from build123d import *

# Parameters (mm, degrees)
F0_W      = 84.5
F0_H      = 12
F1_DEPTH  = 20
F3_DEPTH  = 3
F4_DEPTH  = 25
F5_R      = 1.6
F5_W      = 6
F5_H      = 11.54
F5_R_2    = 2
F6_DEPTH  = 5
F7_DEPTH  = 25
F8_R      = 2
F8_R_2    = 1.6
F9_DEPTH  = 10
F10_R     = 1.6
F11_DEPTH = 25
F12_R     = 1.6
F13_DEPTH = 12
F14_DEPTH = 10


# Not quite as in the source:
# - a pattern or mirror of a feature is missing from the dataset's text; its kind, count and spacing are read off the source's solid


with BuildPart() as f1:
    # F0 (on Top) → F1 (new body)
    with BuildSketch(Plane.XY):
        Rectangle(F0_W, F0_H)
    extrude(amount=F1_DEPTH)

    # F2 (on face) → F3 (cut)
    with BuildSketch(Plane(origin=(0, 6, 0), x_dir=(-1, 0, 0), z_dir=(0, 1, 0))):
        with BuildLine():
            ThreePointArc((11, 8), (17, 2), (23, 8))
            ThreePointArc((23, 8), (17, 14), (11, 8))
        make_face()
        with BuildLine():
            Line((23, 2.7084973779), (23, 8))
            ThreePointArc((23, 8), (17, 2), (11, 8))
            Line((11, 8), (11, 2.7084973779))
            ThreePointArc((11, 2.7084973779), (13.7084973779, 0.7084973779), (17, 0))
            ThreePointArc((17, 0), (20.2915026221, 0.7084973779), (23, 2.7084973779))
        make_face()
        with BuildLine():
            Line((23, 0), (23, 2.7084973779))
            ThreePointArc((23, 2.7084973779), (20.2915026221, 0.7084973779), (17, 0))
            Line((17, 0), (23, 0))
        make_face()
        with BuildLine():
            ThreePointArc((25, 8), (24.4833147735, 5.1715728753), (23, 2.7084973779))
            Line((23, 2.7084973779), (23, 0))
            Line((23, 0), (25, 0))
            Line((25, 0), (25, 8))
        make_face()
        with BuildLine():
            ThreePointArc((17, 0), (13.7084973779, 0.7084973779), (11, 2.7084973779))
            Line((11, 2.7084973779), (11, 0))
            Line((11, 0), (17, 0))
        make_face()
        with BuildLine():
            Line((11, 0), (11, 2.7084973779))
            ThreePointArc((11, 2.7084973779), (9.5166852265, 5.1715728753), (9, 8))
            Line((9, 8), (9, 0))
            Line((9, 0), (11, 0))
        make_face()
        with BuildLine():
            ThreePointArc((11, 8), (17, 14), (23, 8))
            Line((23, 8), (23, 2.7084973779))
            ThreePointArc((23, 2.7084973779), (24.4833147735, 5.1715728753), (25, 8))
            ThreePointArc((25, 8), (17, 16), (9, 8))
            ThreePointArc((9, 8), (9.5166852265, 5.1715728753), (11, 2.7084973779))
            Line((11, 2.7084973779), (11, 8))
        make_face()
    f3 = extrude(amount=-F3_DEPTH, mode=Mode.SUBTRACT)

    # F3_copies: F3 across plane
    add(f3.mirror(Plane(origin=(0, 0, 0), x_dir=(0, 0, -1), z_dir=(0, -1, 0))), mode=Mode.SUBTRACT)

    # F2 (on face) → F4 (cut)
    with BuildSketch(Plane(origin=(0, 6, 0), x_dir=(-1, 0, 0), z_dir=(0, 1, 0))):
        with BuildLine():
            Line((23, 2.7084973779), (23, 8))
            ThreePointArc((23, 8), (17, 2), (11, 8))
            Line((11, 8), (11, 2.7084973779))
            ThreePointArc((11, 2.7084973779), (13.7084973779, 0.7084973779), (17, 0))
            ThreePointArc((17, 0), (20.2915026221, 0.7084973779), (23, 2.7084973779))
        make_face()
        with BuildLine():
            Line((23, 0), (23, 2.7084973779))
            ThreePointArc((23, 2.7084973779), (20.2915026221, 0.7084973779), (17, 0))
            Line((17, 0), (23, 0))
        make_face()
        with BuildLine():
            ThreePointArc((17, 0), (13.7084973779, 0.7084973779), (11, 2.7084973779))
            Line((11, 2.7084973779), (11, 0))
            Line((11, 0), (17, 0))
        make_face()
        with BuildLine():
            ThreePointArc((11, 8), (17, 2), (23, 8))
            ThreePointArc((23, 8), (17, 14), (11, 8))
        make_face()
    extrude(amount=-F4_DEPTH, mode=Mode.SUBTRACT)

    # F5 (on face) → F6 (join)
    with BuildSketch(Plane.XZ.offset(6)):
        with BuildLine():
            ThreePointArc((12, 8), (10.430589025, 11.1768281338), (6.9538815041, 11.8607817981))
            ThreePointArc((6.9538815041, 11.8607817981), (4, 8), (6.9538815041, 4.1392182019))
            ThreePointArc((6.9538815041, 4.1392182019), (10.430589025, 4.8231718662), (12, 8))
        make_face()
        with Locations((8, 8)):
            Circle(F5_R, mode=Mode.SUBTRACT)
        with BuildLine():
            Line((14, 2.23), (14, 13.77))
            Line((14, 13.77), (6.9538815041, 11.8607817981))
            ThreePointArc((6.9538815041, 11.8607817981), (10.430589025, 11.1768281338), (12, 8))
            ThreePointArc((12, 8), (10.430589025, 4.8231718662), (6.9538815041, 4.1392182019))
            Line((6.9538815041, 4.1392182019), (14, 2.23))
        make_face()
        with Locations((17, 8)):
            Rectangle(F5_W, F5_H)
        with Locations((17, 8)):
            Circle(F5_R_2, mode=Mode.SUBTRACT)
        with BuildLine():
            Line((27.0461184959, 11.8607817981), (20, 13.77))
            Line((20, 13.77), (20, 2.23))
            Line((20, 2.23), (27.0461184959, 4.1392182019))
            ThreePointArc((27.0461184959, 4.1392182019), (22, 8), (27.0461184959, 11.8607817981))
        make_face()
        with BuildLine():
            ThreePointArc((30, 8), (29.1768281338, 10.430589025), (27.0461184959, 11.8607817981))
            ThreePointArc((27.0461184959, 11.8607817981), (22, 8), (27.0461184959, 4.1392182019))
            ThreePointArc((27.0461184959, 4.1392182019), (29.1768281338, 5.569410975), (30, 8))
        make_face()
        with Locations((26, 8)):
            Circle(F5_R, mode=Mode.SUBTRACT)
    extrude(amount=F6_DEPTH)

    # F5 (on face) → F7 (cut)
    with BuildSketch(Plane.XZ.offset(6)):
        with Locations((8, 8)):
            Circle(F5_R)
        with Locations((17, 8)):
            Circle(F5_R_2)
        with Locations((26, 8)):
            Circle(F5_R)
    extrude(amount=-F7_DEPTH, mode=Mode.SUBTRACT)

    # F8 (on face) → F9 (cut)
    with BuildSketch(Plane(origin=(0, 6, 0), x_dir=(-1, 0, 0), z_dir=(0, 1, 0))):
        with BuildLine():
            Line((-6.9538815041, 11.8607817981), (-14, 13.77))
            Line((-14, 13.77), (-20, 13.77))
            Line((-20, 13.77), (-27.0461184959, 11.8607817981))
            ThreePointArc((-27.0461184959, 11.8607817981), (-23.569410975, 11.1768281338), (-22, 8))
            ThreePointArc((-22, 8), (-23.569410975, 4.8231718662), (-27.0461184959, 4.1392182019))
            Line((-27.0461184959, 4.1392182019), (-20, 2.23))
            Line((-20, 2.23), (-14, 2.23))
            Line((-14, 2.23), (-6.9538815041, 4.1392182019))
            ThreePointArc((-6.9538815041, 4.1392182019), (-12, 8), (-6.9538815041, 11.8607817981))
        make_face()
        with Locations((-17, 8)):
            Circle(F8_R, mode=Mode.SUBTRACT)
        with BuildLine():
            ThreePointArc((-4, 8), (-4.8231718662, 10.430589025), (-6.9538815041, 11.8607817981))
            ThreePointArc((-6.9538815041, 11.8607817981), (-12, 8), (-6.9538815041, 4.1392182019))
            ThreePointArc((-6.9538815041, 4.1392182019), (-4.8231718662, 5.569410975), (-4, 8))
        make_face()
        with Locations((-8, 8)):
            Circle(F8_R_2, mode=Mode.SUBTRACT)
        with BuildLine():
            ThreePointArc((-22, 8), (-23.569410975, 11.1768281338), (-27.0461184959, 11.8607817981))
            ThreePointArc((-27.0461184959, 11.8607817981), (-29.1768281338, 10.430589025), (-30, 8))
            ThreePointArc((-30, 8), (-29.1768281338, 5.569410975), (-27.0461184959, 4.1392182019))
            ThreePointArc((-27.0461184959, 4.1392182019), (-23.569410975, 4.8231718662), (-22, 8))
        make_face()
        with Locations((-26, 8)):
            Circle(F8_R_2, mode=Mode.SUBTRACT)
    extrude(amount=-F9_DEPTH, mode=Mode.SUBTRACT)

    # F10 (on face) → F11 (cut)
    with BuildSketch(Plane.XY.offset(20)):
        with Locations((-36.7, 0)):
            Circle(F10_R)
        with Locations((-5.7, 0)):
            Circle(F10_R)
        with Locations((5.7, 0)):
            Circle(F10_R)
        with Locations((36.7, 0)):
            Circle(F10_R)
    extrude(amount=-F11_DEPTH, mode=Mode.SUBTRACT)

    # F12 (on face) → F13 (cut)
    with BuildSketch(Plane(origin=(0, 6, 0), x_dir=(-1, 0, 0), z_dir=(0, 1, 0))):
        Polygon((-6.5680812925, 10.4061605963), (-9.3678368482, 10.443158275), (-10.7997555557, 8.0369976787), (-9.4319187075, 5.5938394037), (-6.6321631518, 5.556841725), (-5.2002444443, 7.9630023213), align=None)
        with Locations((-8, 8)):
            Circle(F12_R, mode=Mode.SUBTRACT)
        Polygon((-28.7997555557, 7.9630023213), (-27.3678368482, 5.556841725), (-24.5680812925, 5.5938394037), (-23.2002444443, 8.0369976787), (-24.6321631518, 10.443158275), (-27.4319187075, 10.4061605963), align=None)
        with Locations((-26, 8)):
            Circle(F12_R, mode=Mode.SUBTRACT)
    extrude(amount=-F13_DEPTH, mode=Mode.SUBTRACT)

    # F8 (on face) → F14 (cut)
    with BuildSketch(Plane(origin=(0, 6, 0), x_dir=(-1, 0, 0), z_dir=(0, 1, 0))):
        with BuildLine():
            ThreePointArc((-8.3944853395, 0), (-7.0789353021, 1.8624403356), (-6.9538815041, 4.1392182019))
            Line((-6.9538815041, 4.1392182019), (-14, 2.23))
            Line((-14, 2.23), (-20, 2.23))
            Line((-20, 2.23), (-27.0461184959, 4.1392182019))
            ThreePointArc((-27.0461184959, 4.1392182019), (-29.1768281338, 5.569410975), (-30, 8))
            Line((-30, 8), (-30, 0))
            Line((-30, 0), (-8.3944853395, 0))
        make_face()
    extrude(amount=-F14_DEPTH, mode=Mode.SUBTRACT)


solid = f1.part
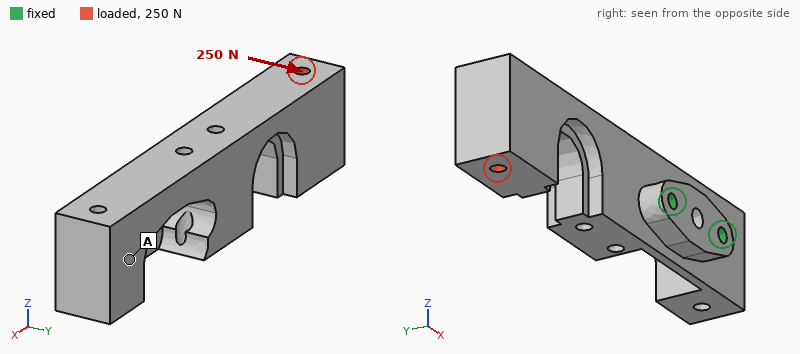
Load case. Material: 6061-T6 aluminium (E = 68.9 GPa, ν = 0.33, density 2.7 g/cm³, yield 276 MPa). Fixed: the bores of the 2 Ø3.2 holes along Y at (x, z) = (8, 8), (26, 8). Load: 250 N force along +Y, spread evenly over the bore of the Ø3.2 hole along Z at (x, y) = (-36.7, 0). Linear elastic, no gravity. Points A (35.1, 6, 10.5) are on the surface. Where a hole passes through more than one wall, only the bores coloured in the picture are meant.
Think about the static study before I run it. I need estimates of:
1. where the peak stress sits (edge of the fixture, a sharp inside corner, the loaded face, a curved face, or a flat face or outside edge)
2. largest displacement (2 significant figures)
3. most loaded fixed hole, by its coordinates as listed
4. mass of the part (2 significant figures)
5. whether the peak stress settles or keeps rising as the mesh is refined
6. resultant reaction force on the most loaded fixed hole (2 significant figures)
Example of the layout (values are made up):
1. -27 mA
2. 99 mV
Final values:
1. a sharp inside corner
2. 0.23 mm
3. (8, 8)
4. 41 g
5. keeps rising
6. 820 N
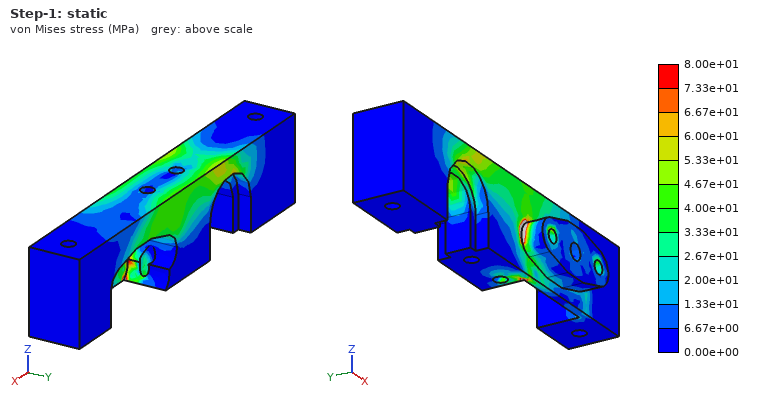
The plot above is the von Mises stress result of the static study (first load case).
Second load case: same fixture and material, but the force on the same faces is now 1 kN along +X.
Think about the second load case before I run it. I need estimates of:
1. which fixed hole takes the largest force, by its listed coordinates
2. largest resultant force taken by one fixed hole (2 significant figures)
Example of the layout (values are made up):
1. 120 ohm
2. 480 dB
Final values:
1. (8, 8)
2. 710 N
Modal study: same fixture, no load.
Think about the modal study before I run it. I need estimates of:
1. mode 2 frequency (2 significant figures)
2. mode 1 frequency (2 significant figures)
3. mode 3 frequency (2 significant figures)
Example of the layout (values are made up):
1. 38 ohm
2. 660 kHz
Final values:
1. 2100 Hz
2. 1600 Hz
3. 4300 Hz
